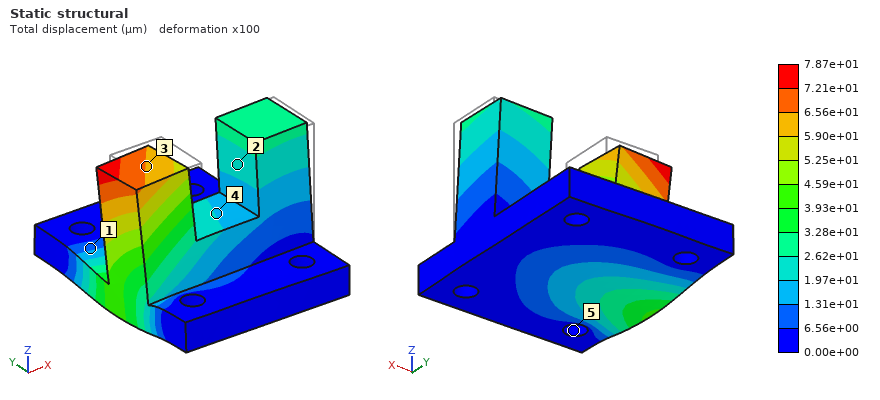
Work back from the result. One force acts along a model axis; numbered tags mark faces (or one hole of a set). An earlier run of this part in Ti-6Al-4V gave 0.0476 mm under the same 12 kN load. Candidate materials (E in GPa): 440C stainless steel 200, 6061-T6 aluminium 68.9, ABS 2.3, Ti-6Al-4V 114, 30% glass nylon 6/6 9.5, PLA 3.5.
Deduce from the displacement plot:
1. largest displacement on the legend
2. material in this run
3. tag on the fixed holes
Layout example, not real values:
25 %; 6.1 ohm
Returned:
7.87e+01 µm; 6061-T6 aluminium; 5
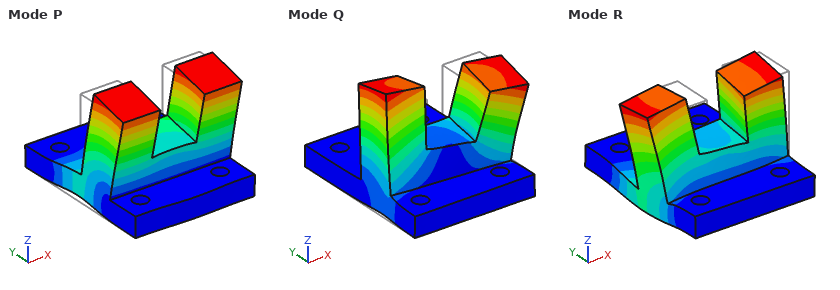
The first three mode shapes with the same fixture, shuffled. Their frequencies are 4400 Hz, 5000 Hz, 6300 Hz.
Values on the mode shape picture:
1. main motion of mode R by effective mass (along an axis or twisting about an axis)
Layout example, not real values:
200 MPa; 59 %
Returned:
along X
